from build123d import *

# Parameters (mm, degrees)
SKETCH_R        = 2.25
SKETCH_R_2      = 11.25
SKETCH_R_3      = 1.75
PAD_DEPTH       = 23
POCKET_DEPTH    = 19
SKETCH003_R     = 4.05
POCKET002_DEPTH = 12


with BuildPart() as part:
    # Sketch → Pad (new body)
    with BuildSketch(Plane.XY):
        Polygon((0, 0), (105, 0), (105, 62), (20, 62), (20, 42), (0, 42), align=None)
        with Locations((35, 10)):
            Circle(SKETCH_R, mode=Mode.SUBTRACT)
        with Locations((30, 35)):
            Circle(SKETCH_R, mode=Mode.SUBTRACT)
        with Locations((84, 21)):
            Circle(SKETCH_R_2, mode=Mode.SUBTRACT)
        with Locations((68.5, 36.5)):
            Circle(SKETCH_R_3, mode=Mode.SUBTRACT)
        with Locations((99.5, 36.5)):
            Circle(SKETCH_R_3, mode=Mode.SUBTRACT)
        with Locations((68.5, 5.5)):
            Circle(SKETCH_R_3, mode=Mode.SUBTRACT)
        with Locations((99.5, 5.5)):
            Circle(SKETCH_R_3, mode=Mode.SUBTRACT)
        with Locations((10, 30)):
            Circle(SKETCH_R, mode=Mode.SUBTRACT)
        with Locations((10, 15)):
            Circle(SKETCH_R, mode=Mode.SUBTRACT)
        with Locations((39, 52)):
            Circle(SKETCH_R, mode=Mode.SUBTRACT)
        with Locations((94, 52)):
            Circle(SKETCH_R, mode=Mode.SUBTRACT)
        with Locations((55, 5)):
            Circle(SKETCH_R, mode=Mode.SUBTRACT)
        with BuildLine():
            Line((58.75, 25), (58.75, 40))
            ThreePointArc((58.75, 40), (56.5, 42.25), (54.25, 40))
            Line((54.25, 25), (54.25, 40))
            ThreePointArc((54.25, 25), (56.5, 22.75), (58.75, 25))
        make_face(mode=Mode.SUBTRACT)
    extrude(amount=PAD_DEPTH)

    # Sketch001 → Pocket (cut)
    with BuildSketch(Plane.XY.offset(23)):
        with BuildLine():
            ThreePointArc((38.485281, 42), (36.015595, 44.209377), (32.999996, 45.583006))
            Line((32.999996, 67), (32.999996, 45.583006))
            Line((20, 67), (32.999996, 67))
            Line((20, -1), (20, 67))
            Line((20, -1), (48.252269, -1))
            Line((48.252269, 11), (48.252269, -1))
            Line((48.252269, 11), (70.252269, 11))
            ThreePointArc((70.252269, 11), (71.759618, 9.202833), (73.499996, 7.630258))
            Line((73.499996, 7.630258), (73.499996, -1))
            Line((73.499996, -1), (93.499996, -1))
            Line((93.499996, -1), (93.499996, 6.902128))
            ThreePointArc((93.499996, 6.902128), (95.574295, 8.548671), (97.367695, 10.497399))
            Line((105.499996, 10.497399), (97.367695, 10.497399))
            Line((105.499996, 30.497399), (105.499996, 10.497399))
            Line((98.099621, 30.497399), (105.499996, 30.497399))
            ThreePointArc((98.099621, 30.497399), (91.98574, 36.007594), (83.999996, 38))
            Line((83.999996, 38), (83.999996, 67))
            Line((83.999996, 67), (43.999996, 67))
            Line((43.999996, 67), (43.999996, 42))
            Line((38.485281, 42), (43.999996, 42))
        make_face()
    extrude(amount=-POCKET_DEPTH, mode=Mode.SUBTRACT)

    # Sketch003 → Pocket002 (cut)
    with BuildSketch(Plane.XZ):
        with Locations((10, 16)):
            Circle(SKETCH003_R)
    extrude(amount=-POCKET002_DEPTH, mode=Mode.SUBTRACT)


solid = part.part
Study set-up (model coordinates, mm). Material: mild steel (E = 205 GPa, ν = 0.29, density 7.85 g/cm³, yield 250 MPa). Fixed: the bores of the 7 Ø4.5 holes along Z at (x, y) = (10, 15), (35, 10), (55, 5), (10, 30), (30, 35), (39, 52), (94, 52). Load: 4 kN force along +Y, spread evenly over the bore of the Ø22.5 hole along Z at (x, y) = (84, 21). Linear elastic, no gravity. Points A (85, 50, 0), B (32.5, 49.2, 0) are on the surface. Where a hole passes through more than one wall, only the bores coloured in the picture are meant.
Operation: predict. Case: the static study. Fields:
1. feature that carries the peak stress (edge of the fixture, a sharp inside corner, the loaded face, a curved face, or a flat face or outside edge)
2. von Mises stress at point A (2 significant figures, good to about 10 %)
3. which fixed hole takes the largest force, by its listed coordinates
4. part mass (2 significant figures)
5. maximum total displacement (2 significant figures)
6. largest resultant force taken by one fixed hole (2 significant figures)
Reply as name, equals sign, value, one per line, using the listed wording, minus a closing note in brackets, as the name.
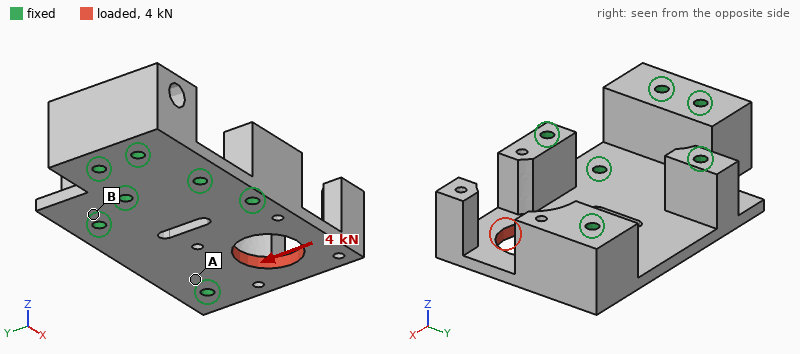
feature that carries the peak stress = the loaded face
von Mises stress at point A = 9.5 MPa
which fixed hole takes the largest force, by its listed coordinates = (94, 52)
part mass = 450 g
maximum total displacement = 7.3 µm
largest resultant force taken by one fixed hole = 2.5 kN
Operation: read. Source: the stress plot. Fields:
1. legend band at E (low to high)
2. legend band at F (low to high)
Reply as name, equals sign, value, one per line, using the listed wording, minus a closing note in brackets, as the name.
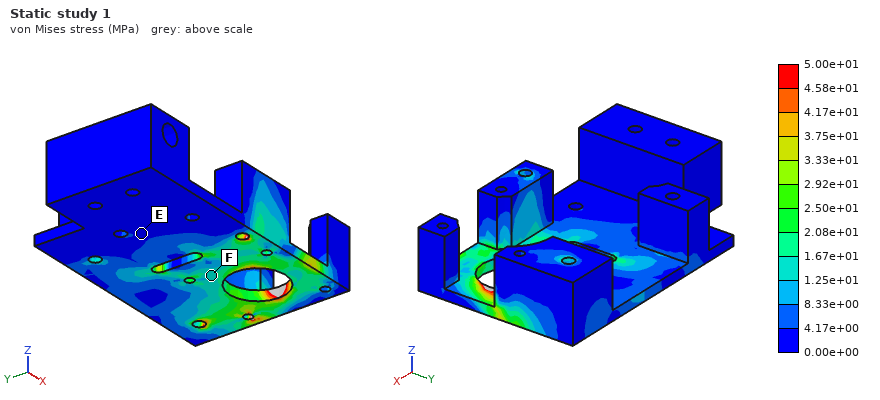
legend band at E = 0.00e+00 to 4.17e+00 MPa
legend band at F = 1.25e+01 to 1.67e+01 MPa
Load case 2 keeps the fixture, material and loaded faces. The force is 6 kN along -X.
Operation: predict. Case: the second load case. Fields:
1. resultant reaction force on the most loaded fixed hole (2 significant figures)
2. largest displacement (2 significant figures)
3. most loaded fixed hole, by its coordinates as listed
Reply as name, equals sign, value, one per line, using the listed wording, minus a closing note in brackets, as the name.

resultant reaction force on the most loaded fixed hole = 2.6 kN
largest displacement = 11 µm
most loaded fixed hole, by its coordinates as listed = (55, 5)
